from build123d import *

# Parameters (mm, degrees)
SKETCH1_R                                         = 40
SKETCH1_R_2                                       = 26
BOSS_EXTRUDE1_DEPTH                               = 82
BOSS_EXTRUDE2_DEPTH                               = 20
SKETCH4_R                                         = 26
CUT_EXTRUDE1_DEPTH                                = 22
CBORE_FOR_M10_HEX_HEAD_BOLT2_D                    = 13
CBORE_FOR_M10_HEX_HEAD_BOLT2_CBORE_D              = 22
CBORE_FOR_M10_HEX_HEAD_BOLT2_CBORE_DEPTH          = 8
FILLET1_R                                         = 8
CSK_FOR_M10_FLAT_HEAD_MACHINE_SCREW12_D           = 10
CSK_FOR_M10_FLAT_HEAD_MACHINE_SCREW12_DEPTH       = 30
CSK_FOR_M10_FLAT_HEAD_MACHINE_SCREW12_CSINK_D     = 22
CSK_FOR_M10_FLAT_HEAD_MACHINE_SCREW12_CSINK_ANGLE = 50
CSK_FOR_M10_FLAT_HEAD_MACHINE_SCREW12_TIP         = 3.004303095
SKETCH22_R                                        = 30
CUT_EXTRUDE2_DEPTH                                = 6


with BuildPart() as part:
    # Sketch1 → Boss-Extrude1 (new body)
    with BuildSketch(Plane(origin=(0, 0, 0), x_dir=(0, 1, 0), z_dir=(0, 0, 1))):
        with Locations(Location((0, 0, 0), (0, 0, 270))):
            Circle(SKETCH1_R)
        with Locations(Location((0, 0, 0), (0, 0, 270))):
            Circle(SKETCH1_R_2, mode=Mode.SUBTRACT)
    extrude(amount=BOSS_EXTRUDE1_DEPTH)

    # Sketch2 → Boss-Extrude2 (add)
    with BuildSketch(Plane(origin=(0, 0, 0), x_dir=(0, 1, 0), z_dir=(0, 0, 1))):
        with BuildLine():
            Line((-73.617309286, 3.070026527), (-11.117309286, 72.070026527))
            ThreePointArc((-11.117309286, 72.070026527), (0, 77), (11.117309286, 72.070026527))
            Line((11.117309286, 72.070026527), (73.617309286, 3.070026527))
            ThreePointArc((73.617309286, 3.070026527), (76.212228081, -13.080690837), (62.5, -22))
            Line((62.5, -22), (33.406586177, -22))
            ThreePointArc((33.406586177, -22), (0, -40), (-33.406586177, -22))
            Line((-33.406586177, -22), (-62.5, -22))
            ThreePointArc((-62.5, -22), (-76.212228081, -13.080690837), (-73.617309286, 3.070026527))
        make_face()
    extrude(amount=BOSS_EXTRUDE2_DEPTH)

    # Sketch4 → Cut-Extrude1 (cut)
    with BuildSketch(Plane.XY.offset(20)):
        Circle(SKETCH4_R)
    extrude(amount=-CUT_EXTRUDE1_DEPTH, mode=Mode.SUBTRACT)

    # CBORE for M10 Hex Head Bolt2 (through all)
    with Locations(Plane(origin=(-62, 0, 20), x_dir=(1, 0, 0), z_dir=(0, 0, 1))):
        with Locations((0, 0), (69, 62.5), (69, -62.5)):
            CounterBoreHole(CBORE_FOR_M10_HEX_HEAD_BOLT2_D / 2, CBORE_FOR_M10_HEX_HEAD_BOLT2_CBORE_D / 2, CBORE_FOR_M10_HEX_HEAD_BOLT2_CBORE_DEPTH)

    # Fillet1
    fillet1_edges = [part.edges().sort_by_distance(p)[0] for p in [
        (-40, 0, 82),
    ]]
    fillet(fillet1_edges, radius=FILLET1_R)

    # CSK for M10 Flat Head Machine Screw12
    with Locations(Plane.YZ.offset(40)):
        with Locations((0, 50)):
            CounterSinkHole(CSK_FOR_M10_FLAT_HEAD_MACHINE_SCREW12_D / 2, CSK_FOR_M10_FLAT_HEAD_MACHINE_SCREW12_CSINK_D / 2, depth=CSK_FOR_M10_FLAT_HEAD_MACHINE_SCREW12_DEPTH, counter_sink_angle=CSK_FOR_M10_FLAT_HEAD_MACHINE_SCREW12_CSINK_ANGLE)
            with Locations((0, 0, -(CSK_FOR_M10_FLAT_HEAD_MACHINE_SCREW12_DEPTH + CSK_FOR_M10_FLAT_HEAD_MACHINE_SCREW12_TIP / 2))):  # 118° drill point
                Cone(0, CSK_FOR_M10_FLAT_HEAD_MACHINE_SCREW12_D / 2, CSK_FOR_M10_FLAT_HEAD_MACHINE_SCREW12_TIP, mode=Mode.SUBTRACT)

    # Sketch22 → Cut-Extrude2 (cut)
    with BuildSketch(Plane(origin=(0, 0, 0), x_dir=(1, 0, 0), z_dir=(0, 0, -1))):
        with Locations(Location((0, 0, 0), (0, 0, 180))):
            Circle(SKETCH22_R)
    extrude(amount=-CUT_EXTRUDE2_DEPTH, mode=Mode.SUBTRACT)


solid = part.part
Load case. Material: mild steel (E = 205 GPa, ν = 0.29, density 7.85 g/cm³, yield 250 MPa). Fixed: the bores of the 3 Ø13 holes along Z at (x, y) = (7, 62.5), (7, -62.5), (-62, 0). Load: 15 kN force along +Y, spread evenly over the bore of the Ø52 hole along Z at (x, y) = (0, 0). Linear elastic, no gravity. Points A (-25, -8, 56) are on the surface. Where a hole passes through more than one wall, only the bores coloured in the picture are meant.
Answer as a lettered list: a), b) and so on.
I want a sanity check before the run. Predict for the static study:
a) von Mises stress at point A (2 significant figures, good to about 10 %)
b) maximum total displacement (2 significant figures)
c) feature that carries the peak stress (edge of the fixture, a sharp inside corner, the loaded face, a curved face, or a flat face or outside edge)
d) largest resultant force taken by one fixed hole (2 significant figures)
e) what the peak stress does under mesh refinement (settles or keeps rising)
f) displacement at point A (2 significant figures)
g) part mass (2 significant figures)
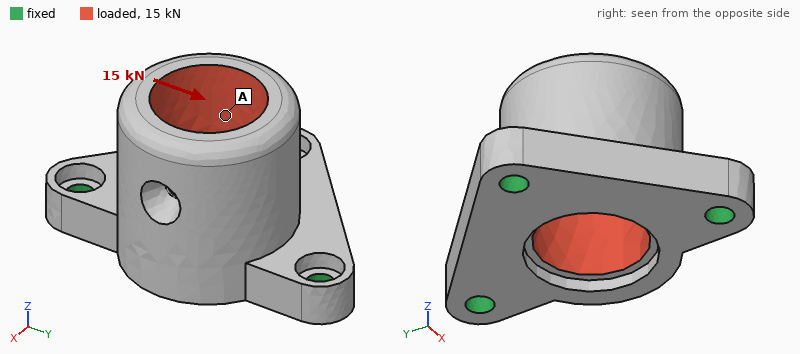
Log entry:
a) 7.5 MPa
b) 14 µm
c) edge of the fixture
d) 8.3 kN
e) keeps rising
f) 9.0 µm
g) 2.5 kg
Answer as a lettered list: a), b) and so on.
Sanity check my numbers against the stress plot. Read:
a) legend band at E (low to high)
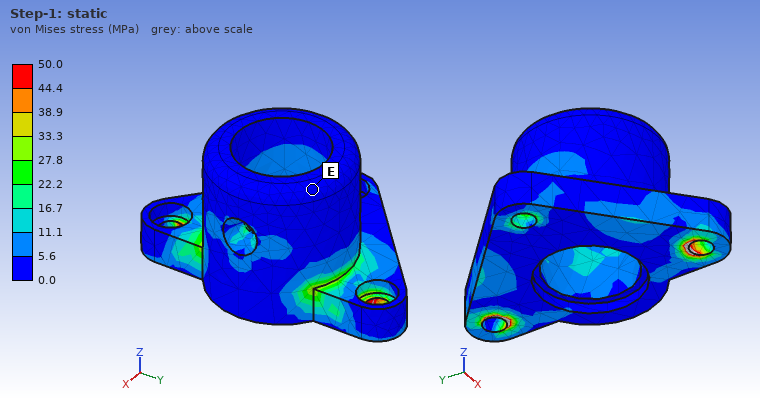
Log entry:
a) 0.0 to 5.6 MPa
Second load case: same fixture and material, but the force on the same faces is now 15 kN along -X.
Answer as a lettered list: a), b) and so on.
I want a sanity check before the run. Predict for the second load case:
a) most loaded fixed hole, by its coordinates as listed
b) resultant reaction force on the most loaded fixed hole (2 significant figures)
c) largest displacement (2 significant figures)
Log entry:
a) (-62, 0)
b) 12 kN
c) 37 µm
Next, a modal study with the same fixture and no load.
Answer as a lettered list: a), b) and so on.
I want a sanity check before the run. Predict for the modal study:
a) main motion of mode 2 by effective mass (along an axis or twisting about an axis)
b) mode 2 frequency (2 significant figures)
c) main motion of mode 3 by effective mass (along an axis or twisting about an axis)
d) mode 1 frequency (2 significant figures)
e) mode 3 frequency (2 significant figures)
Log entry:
a) along Y
b) 4500 Hz
c) along Z
d) 2800 Hz
e) 5500 Hz
